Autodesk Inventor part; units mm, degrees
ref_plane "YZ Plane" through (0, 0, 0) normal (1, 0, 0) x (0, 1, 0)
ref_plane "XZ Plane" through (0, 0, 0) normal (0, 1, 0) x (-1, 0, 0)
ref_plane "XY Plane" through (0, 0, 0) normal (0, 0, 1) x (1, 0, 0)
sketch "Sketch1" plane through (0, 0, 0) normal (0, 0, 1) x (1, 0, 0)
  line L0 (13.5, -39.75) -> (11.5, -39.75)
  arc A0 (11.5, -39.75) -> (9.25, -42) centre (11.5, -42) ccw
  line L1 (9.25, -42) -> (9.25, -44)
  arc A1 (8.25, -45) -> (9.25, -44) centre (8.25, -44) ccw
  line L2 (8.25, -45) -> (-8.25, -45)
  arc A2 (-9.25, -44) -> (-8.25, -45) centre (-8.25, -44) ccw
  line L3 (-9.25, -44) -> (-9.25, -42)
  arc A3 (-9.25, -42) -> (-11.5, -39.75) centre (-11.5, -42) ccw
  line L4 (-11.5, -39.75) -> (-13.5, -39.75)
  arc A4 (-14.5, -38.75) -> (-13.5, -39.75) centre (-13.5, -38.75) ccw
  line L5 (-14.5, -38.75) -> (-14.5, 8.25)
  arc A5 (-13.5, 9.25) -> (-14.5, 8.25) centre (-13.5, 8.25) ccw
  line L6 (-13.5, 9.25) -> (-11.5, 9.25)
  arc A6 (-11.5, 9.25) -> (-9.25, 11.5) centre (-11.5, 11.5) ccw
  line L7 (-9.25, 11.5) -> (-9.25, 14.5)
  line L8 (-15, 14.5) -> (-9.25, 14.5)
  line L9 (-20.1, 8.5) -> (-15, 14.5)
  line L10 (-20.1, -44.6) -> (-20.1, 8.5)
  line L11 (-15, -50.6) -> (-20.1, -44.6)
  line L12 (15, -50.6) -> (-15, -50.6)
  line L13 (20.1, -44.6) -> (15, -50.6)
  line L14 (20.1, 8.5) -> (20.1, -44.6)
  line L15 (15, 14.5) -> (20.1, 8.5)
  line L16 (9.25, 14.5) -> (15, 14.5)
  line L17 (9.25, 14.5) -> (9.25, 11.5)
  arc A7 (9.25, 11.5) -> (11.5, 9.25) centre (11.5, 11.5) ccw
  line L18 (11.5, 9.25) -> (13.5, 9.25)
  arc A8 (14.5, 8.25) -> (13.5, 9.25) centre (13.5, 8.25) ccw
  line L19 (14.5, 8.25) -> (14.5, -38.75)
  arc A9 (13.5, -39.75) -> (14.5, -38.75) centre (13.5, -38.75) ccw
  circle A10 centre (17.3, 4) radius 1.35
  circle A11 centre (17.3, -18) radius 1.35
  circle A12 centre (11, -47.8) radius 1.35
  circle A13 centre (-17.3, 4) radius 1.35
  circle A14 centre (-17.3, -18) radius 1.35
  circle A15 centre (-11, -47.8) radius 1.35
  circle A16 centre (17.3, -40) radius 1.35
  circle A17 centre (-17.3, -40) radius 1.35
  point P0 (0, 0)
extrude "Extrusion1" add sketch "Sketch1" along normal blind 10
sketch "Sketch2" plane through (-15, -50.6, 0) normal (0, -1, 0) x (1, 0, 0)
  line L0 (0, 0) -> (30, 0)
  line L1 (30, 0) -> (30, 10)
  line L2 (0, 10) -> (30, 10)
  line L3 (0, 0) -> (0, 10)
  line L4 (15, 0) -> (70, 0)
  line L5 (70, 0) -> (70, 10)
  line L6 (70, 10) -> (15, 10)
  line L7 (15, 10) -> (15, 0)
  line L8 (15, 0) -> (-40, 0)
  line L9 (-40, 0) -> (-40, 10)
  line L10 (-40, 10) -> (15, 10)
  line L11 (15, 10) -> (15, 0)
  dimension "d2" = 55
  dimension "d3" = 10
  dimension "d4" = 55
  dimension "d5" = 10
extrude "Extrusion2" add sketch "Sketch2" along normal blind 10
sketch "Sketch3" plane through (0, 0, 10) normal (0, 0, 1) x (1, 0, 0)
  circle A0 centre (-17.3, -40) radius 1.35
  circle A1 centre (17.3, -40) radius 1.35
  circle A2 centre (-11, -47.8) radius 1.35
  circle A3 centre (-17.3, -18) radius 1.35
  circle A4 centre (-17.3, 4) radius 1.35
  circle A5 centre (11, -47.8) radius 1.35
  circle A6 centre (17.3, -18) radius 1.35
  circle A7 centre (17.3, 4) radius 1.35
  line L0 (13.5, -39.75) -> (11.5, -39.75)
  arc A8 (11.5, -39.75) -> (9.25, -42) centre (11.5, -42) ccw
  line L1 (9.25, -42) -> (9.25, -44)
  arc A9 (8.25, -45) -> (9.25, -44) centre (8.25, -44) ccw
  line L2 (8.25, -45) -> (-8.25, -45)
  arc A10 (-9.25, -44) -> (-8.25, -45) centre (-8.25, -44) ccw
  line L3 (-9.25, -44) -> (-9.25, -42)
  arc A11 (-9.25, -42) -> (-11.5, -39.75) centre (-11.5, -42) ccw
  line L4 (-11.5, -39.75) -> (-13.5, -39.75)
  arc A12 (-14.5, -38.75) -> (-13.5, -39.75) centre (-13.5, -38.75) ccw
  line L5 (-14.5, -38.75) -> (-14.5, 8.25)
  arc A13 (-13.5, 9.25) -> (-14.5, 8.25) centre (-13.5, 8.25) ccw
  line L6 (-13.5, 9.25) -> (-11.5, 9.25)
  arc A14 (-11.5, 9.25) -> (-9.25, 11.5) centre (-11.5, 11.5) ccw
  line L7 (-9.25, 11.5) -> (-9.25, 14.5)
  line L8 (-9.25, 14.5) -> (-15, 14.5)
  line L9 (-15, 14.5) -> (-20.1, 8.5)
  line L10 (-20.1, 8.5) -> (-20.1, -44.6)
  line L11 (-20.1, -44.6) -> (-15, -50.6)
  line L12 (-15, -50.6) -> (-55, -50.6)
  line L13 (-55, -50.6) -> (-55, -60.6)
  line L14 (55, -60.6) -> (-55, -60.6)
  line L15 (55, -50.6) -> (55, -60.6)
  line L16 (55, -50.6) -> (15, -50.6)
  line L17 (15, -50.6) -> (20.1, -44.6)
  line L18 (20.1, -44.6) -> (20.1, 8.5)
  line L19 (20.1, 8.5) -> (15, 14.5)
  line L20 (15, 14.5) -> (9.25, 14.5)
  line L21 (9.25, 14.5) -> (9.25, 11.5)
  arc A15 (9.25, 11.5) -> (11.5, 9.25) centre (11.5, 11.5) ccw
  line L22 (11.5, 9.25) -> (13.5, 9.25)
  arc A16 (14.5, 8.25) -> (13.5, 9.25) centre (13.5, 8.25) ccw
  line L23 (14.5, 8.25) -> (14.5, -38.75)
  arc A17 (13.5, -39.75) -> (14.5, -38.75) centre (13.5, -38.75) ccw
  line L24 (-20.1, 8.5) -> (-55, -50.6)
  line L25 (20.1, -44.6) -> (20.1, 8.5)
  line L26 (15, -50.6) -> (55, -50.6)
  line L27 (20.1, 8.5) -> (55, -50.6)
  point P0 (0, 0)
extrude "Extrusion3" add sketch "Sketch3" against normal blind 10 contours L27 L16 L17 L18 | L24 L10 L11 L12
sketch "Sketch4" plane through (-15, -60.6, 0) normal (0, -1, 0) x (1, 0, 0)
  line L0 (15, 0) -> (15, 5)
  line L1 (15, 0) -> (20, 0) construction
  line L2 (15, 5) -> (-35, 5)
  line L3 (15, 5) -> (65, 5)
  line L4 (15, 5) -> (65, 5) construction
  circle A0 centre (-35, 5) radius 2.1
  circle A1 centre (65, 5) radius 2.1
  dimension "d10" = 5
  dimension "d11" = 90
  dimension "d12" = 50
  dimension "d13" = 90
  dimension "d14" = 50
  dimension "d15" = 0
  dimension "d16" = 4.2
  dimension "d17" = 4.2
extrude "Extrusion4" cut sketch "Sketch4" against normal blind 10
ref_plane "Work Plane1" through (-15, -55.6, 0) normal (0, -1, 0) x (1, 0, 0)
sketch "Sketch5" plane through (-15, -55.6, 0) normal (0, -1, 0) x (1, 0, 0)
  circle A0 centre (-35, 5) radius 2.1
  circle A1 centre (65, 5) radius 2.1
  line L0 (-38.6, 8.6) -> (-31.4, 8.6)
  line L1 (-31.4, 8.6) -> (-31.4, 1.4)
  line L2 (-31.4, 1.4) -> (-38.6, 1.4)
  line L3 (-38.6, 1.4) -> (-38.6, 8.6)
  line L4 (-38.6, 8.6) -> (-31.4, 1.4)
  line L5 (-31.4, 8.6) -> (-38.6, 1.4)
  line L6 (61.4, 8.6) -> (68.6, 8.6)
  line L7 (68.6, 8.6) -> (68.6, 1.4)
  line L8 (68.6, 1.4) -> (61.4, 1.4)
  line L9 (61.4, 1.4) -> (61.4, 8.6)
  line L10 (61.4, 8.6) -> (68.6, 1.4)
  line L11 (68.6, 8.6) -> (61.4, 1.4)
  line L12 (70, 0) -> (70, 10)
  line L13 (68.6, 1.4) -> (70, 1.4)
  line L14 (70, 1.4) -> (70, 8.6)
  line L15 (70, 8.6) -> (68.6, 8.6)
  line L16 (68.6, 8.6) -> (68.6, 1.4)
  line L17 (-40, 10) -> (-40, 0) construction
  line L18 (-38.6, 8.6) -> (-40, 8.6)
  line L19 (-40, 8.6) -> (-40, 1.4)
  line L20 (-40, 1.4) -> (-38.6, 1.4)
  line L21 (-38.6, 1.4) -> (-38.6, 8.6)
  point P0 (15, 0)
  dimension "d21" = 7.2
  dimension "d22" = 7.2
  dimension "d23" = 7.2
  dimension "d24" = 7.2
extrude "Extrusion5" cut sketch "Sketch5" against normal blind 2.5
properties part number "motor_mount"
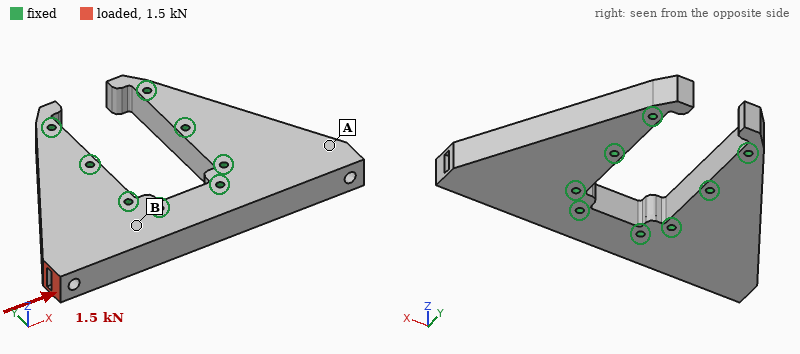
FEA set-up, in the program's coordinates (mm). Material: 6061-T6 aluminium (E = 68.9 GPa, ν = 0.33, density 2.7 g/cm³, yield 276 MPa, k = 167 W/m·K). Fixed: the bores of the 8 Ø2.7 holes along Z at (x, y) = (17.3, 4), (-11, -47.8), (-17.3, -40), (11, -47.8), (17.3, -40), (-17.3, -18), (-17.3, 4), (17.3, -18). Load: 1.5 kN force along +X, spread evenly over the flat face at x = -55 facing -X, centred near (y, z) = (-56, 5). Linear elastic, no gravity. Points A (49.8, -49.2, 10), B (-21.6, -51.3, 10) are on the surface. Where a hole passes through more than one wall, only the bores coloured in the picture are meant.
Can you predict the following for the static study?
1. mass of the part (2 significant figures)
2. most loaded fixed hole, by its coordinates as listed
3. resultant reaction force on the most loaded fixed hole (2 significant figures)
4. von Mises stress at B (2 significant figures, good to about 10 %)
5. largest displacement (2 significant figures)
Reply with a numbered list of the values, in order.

1. 110 g
2. (-11, -47.8)
3. 910 N
4. 8.7 MPa
5. 16 µm
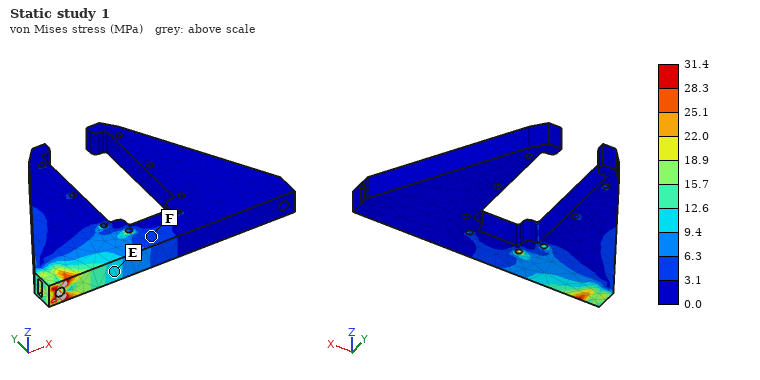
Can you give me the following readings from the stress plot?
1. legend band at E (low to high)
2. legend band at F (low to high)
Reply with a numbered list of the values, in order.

1. 9.4 to 12.6 MPa
2. 3.1 to 6.3 MPa
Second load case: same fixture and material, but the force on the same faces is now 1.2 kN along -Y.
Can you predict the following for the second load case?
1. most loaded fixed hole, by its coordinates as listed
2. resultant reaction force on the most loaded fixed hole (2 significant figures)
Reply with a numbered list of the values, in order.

1. (-17.3, -18)
2. 1.0 kN
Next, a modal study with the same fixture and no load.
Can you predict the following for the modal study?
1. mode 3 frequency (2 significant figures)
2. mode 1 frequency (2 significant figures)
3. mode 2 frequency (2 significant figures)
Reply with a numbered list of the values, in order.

1. 15 kHz
2. 6100 Hz
3. 6100 Hz
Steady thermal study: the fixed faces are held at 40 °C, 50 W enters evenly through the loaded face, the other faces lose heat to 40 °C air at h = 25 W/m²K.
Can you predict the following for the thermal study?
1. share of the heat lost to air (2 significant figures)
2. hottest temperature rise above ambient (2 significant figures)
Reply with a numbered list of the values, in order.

1. 3.7 %
2. 74 K
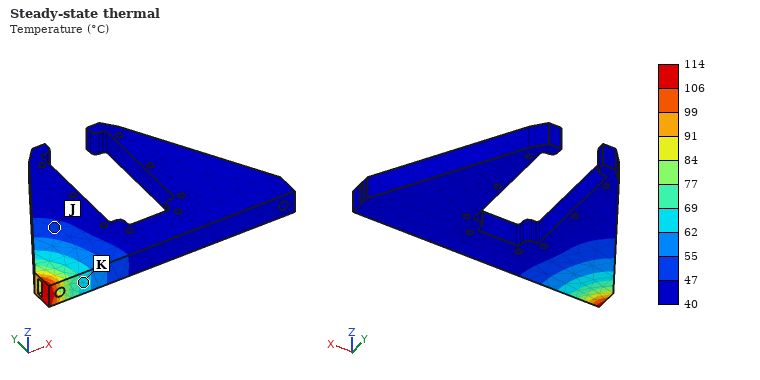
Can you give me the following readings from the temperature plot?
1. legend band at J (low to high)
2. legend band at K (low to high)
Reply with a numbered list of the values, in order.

1. 47 to 55 °C
2. 62 to 69 °C
